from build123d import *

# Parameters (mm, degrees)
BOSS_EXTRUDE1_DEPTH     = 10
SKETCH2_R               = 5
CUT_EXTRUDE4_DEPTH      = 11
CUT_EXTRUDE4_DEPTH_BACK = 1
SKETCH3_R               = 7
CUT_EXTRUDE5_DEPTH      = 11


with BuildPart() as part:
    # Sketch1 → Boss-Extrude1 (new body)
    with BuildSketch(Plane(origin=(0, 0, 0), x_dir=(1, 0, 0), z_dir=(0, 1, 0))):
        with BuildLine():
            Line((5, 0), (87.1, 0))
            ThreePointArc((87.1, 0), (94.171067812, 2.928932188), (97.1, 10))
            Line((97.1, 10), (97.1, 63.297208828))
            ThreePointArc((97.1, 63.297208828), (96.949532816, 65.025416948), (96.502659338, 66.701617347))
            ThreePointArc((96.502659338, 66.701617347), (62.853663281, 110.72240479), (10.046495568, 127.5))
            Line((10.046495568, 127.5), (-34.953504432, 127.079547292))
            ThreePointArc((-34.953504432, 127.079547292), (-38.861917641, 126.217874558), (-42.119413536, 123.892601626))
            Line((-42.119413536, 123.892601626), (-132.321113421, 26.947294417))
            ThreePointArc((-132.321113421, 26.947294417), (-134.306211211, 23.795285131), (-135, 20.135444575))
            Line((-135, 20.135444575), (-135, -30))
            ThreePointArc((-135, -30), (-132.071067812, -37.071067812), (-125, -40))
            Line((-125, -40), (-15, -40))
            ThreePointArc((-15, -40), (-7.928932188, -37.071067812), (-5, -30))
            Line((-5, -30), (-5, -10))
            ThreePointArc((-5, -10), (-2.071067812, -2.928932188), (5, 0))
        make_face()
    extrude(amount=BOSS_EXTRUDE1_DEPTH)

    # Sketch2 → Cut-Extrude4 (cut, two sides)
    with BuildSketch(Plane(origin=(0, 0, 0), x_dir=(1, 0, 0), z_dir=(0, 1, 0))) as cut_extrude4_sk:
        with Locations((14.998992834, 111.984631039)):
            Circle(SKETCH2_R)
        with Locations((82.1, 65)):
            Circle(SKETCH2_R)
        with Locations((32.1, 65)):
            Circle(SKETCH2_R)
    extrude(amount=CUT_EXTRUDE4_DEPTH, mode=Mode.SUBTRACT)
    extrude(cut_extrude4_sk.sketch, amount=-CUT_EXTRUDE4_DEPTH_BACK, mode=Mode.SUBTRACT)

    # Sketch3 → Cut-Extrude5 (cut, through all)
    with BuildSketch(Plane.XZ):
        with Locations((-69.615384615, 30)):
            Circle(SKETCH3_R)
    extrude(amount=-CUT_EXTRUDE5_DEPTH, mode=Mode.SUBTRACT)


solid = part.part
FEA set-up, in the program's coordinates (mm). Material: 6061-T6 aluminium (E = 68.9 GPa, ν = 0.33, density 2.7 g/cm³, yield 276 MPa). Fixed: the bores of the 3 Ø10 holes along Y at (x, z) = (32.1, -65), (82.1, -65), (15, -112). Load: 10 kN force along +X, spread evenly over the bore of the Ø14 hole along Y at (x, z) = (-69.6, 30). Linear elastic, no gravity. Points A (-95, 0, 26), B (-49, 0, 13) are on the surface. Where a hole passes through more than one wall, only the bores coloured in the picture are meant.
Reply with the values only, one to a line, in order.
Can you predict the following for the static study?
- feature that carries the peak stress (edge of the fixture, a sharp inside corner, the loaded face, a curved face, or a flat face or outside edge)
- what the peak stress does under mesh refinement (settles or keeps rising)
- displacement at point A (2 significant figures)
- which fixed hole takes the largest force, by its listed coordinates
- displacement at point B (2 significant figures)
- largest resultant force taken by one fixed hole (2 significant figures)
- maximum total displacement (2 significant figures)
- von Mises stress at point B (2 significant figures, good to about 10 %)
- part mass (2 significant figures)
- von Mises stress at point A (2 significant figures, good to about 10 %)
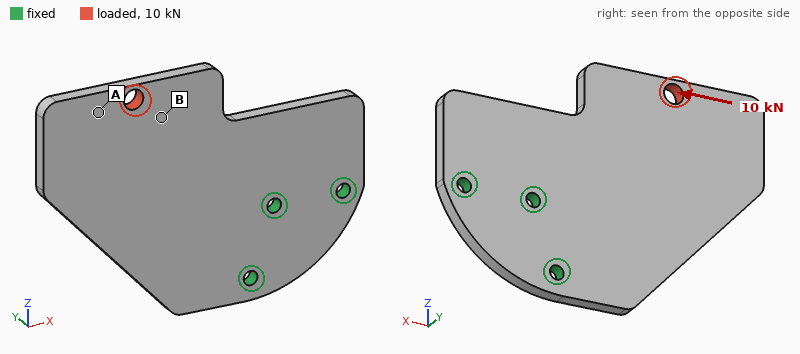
edge of the fixture
keeps rising
0.17 mm
(32.1, -65)
0.12 mm
13 kN
0.21 mm
24 MPa
750 g
10 MPa
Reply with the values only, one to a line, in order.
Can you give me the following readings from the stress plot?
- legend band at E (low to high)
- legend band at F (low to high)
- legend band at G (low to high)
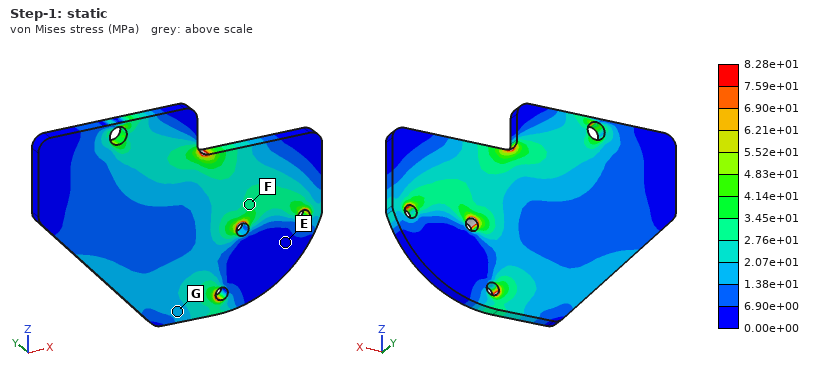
0.00e+00 to 6.90e+00 MPa
2.76e+01 to 3.45e+01 MPa
1.38e+01 to 2.07e+01 MPa
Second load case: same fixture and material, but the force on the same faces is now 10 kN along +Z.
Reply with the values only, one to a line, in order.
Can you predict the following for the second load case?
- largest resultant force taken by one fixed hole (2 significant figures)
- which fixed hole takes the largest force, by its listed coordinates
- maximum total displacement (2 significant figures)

14 kN
(15, -112)
0.17 mm
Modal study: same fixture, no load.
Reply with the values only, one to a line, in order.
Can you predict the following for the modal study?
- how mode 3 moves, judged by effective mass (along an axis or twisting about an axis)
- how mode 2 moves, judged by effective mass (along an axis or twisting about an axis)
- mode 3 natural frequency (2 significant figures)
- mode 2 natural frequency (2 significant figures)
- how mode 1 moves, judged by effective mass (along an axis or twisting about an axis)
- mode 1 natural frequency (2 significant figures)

along Y
twisting about X
1400 Hz
920 Hz
along Y
290 Hz
